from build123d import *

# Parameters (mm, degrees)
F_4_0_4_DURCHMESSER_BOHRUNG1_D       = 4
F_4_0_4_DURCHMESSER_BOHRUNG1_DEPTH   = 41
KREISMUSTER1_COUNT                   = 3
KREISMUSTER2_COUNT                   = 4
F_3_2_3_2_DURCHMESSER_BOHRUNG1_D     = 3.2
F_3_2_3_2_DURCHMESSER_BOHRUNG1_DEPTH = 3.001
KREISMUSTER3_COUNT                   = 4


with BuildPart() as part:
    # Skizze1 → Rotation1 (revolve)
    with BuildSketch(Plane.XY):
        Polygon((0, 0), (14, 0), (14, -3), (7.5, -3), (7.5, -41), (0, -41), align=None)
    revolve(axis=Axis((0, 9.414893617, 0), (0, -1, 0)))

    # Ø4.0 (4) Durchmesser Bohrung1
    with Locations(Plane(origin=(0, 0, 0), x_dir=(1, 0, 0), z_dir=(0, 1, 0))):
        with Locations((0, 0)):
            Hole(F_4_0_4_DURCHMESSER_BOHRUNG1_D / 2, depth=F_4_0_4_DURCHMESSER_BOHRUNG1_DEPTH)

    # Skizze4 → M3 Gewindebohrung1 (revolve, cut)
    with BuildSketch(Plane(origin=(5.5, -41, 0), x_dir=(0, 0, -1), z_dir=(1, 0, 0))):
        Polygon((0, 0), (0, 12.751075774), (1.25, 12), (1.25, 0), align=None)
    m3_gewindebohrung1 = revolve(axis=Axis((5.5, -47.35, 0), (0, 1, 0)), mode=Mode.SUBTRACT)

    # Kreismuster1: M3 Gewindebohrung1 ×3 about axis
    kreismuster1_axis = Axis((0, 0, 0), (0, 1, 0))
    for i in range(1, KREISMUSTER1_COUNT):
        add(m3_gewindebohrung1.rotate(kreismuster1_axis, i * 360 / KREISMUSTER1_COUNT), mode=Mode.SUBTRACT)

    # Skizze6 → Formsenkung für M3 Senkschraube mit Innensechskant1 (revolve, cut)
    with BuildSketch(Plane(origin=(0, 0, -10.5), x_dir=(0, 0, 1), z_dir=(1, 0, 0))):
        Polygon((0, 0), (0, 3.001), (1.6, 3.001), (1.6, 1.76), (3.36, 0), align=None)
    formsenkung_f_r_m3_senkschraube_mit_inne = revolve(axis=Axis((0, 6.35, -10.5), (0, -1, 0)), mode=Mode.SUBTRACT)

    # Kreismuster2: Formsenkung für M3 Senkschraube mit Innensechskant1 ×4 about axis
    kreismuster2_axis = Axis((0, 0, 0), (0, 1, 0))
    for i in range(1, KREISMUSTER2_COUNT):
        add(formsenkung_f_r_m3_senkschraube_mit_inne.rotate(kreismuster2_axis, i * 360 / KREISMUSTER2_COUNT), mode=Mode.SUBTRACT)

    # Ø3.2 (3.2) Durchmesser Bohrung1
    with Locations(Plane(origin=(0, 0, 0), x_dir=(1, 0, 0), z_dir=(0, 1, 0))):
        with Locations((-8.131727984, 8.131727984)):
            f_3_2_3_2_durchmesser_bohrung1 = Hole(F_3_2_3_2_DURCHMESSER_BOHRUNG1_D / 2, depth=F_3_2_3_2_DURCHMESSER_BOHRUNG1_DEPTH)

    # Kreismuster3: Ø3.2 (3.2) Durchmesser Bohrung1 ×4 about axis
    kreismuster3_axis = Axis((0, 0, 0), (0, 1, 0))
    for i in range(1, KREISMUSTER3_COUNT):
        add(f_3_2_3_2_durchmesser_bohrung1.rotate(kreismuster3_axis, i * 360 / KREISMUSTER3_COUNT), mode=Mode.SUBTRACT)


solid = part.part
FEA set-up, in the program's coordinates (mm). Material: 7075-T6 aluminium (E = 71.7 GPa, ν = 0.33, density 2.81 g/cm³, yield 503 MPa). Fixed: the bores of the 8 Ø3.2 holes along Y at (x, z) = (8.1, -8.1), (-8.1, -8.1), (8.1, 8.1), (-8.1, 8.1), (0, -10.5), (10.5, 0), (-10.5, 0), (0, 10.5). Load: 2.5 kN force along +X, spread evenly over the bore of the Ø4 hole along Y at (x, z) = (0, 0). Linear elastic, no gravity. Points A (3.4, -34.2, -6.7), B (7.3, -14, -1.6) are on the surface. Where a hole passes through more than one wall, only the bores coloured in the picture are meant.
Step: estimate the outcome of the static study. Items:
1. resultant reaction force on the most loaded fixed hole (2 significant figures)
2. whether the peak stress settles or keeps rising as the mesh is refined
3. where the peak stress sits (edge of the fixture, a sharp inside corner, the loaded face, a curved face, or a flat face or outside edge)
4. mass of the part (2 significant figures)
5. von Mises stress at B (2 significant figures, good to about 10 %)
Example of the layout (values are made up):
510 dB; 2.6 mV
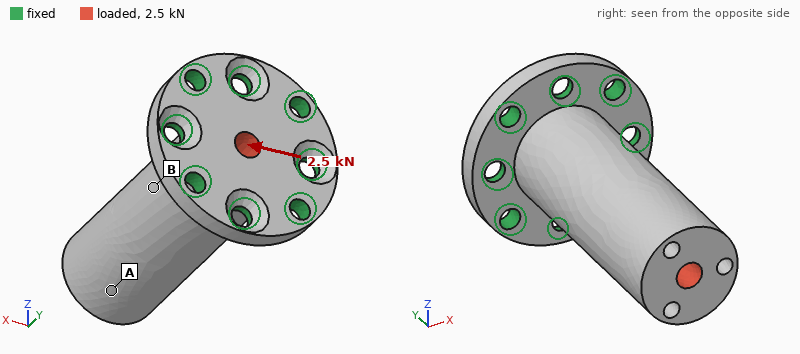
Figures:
1.3 kN; keeps rising; edge of the fixture; 21 g; 65 MPa
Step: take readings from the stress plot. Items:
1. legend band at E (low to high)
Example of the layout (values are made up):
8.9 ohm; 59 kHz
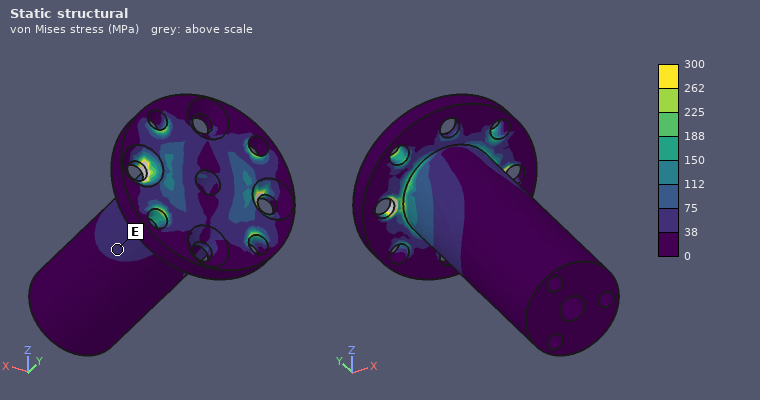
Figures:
38 to 75 MPa
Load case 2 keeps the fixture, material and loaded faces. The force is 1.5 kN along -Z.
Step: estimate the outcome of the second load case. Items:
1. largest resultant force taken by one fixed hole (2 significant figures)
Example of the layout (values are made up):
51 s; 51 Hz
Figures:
800 N
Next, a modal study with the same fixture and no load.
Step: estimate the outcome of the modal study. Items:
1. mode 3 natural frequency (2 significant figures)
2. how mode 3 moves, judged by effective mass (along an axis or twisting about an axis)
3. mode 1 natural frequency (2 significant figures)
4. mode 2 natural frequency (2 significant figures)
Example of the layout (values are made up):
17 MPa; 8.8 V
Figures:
20 kHz; twisting about Y; 5300 Hz; 5300 Hz
